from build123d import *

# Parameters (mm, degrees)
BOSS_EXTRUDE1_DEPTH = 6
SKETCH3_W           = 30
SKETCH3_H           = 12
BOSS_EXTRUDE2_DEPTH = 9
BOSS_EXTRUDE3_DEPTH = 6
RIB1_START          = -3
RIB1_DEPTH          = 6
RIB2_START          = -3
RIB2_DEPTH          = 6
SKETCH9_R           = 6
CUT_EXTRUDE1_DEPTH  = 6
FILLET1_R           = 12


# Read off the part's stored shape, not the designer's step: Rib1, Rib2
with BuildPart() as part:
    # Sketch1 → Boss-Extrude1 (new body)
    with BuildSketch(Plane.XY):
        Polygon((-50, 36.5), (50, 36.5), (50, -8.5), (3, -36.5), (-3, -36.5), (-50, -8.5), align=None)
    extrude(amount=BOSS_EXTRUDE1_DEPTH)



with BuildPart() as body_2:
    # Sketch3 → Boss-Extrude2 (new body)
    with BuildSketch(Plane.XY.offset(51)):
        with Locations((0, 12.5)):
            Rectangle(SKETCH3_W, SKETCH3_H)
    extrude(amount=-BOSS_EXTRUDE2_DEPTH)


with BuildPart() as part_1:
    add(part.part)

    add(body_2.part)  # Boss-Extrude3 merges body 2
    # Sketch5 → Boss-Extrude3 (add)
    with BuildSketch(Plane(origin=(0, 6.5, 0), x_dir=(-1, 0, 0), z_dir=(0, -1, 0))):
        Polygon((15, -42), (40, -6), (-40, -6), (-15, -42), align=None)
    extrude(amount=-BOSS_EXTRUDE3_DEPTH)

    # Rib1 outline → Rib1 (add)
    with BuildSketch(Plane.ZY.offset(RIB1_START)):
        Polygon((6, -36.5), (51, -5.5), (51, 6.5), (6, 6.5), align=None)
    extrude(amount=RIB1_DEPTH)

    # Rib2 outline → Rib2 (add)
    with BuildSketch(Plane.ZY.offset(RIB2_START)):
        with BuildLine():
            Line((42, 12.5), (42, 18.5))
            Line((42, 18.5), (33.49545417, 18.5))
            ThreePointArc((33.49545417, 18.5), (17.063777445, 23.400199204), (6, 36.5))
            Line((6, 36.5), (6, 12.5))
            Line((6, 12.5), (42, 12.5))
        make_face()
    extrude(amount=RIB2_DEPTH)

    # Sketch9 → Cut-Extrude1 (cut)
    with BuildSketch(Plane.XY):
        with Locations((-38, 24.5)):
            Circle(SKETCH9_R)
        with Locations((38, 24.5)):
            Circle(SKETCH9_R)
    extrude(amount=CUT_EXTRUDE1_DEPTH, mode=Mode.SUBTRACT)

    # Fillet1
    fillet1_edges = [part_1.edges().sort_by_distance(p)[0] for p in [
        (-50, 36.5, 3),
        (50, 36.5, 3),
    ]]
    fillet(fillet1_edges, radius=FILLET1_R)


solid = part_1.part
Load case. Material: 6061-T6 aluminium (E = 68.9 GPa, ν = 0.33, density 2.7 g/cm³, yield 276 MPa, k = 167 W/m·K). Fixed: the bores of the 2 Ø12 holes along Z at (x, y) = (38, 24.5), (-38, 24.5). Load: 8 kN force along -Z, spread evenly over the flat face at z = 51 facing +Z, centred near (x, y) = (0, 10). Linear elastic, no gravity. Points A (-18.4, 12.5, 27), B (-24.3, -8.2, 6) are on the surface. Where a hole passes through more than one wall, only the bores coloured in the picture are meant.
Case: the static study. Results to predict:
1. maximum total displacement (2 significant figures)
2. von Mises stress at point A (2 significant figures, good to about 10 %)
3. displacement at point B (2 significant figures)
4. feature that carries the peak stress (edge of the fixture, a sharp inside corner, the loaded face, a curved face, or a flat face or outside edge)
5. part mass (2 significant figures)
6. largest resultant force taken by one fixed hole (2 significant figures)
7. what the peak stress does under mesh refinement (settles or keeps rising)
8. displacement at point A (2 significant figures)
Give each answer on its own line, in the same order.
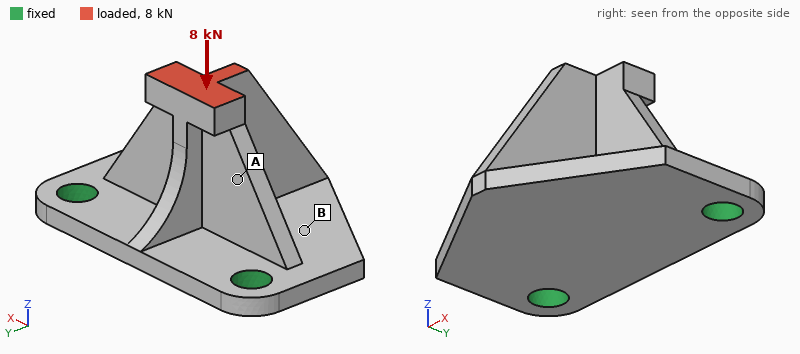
0.31 mm
47 MPa
0.17 mm
edge of the fixture
160 g
4.3 kN
keeps rising
0.14 mm
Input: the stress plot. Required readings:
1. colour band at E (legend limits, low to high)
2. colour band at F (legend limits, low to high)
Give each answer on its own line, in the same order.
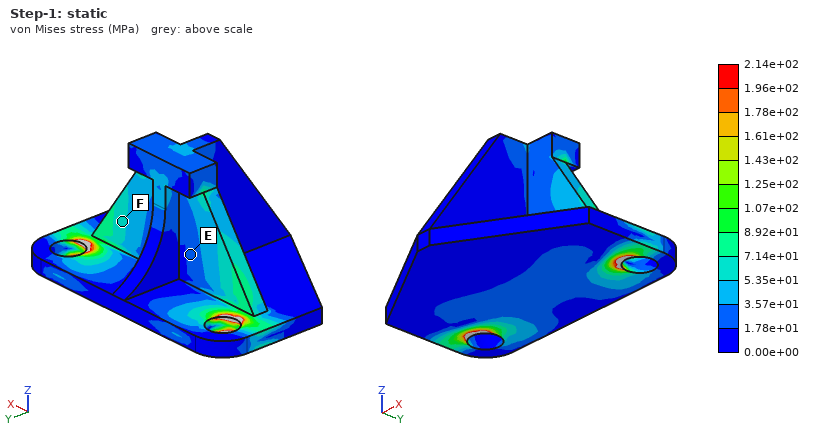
1.78e+01 to 3.57e+01 MPa
5.35e+01 to 7.14e+01 MPa
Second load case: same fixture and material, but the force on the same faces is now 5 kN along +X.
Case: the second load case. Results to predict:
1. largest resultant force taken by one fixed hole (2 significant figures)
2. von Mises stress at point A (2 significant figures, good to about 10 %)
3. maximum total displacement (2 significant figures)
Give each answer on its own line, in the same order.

4.3 kN
54 MPa
0.13 mm
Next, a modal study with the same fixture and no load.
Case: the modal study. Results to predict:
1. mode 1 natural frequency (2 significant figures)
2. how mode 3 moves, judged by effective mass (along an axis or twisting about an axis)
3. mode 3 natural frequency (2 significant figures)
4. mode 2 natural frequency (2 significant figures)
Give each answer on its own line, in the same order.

1500 Hz
along Z
5400 Hz
4900 Hz
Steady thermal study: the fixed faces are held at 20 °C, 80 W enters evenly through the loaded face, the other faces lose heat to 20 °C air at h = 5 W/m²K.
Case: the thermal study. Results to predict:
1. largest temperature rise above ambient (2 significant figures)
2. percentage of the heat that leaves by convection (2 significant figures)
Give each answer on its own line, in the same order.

72 K
3.2 %
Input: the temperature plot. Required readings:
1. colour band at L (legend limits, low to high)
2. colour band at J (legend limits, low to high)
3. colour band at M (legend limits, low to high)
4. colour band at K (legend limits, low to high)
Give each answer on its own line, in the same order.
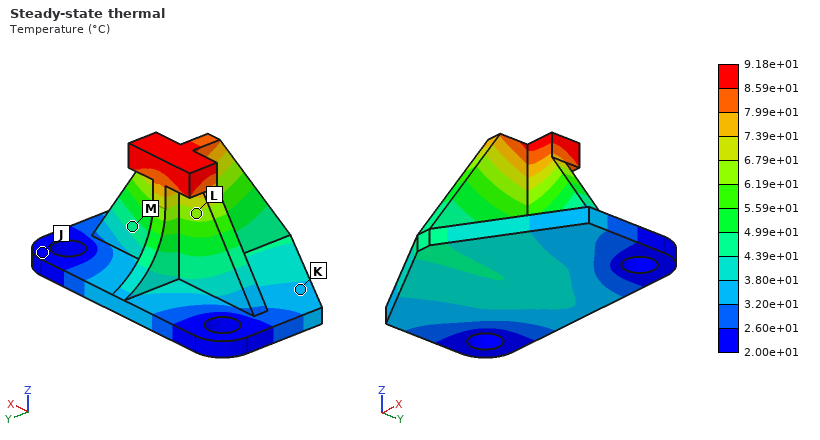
6.19e+01 to 6.79e+01 °C
2.00e+01 to 2.60e+01 °C
4.39e+01 to 4.99e+01 °C
3.20e+01 to 3.80e+01 °C
